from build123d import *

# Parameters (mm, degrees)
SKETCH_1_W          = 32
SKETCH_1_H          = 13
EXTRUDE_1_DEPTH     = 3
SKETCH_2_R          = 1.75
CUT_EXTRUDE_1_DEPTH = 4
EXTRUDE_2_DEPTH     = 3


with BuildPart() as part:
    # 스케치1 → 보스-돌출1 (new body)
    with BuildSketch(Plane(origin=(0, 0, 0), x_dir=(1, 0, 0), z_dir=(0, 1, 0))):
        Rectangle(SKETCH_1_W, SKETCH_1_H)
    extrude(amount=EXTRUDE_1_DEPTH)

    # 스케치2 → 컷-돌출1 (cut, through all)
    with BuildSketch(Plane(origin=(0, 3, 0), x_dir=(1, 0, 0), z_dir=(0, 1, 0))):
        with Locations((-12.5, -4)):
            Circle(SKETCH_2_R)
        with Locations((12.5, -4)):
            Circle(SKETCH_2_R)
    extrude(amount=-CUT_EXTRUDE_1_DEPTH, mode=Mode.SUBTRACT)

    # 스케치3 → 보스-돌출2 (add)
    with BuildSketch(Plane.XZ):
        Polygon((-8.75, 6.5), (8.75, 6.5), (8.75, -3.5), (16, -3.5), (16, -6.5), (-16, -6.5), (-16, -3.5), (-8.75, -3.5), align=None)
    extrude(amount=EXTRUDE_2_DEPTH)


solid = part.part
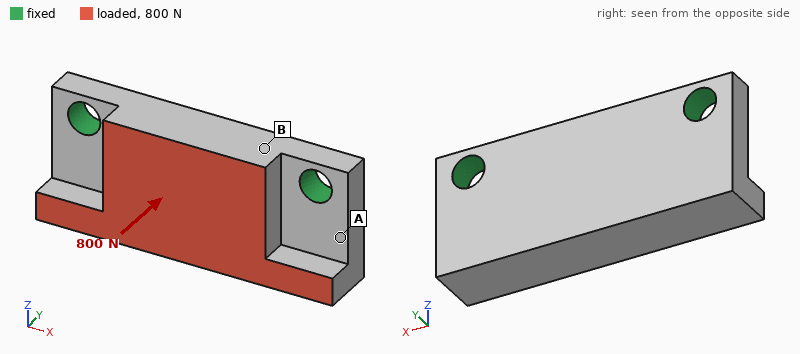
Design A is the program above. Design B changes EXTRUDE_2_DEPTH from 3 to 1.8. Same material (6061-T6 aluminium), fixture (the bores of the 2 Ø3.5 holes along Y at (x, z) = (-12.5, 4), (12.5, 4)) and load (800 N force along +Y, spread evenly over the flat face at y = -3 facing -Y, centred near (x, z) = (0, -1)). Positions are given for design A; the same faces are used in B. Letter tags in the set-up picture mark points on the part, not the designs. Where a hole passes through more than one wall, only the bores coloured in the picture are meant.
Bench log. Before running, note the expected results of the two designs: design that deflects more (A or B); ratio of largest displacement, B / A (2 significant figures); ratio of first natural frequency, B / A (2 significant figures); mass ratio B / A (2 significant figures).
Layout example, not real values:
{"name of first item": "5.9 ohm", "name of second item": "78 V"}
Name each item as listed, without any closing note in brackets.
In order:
{"design that deflects more": "B", "ratio of largest displacement, B / A": "1.1", "ratio of first natural frequency, B / A": "1.1", "mass ratio B / A": "0.84"}
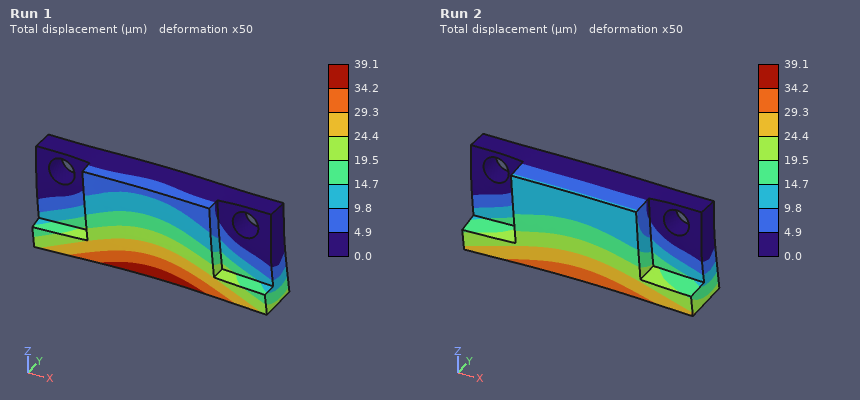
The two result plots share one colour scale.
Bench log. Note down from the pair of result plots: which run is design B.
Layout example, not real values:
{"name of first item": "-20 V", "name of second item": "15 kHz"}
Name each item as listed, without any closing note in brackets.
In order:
{"which run is design B": "Run 1"}
